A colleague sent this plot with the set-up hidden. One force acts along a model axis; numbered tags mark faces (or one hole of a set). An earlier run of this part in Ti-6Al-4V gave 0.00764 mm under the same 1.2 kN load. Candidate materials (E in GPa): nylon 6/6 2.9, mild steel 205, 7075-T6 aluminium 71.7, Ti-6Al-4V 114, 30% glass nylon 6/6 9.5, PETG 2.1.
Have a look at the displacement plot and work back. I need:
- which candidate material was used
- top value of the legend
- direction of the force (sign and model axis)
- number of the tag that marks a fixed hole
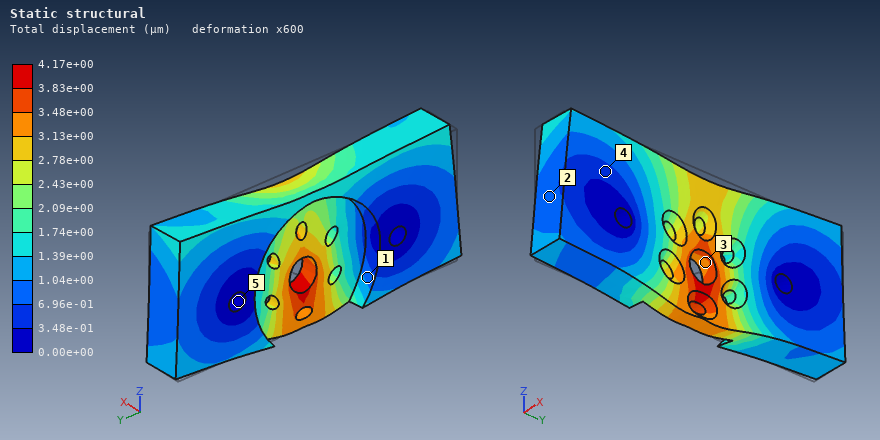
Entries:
mild steel
4.17e+00 µm
-Z
5
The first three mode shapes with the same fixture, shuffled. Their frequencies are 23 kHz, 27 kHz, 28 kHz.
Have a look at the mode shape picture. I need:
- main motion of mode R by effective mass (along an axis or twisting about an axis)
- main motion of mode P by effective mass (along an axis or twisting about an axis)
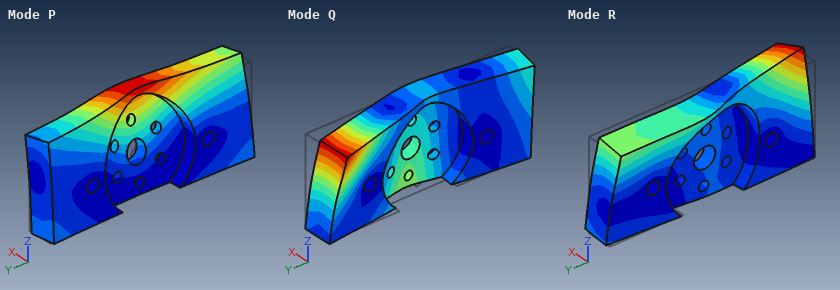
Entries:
twisting about Z
along X
